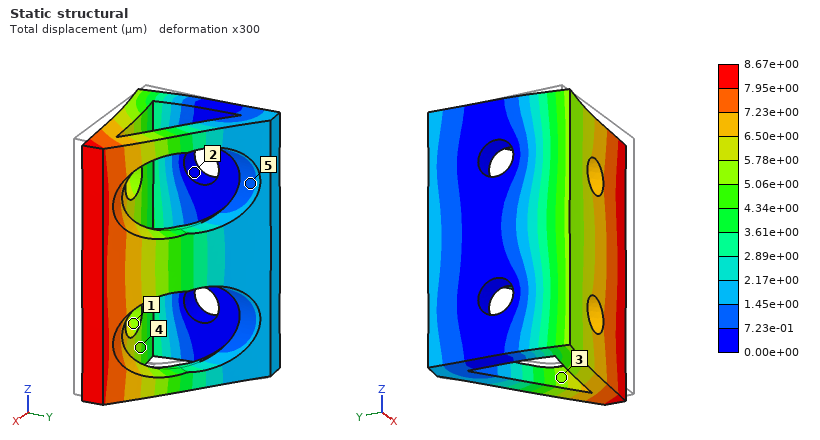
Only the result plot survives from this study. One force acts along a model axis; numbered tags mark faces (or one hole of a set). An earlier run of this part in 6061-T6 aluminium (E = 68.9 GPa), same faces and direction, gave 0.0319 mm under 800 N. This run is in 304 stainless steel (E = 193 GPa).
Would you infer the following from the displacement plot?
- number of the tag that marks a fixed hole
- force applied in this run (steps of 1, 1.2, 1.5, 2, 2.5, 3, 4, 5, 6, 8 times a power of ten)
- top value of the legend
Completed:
2
600 N
8.67e+00 µm
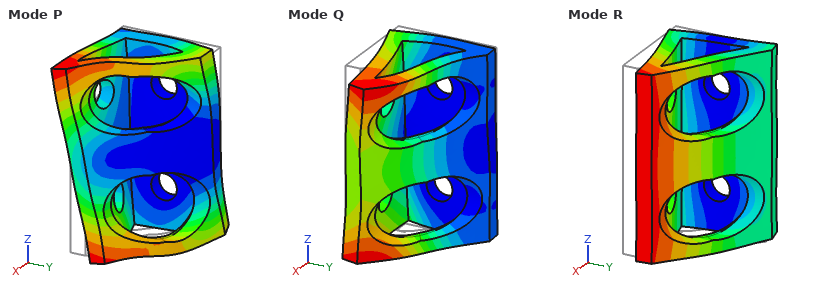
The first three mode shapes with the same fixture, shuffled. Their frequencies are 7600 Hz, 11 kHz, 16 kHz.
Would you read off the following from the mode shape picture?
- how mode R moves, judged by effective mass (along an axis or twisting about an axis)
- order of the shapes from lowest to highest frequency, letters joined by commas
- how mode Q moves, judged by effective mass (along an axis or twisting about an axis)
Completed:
along Y
R, Q, P
along Z
